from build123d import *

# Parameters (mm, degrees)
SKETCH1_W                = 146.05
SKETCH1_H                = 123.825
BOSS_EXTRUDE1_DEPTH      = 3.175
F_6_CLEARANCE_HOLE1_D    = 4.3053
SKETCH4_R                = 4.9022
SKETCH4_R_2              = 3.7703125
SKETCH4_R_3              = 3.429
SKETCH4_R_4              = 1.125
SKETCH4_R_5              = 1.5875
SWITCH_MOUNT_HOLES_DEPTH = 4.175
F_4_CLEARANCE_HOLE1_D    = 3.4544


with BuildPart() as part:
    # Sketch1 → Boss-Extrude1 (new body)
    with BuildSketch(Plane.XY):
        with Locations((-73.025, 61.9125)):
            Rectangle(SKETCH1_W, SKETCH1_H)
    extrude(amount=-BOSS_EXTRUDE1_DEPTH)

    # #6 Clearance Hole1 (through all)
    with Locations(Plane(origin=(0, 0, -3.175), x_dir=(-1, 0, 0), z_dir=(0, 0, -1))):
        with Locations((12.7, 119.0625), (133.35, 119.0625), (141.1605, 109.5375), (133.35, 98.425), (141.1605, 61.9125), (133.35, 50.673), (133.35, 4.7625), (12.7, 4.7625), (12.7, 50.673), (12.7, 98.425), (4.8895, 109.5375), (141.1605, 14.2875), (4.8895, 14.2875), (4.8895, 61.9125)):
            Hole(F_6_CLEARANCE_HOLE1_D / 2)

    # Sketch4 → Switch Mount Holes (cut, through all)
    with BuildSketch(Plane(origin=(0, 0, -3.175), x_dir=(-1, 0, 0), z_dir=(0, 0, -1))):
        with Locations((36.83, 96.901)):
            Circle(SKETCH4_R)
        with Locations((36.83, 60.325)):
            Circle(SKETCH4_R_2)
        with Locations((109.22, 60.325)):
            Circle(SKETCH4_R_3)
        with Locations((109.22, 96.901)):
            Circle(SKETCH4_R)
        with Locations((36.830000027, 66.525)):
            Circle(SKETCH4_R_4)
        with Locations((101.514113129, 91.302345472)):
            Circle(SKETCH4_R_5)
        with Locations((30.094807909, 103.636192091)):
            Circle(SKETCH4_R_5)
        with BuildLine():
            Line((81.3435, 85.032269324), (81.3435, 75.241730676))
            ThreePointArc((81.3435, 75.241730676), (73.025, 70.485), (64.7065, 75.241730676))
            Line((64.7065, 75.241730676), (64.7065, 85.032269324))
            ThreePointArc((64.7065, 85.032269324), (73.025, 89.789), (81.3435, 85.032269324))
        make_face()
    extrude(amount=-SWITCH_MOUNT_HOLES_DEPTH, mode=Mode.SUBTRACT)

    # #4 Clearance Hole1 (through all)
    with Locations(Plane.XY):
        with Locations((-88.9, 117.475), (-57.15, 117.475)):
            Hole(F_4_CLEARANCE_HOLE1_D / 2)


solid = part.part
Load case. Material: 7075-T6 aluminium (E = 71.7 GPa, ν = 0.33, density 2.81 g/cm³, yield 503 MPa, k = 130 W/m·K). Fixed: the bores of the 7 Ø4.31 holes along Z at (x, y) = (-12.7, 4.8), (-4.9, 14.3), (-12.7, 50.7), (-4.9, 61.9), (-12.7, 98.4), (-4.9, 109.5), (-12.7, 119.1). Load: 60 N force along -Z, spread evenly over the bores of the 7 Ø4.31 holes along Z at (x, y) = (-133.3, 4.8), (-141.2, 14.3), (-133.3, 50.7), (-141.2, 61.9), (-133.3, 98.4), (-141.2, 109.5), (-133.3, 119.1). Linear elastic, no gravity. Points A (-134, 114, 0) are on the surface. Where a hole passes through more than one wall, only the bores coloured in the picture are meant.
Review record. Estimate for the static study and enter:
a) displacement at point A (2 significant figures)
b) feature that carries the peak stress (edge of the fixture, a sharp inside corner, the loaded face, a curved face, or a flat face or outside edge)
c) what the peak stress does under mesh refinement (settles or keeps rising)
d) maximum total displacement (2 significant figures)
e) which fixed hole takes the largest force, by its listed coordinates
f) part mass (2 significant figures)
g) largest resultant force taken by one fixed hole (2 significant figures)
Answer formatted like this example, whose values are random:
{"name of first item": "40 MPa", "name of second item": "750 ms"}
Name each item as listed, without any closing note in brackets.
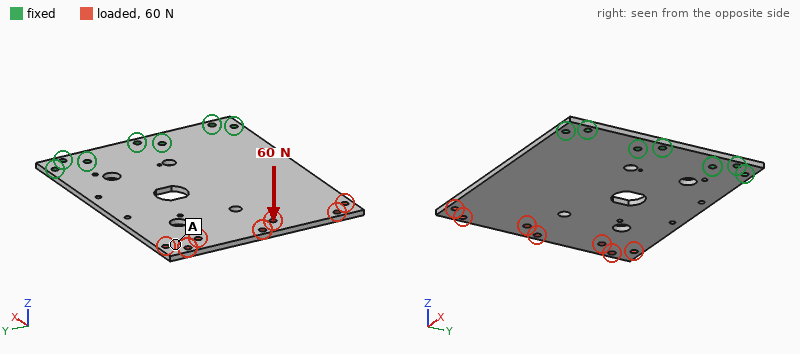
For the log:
{"displacement at point A": "1.7 mm", "feature that carries the peak stress": "edge of the fixture", "what the peak stress does under mesh refinement": "keeps rising", "maximum total displacement": "1.9 mm", "which fixed hole takes the largest force, by its listed coordinates": "(-12.7, 50.7)", "part mass": "150 g", "largest resultant force taken by one fixed hole": "120 N"}
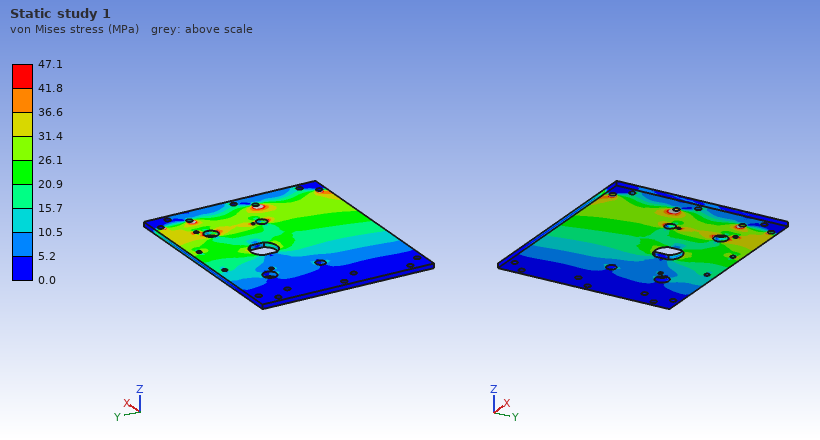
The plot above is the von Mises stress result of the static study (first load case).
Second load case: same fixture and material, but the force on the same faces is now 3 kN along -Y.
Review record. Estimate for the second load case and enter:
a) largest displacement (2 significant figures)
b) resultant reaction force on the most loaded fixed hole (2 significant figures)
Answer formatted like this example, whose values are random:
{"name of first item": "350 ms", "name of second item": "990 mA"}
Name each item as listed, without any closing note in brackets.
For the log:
{"largest displacement": "0.13 mm", "resultant reaction force on the most loaded fixed hole": "2.3 kN"}
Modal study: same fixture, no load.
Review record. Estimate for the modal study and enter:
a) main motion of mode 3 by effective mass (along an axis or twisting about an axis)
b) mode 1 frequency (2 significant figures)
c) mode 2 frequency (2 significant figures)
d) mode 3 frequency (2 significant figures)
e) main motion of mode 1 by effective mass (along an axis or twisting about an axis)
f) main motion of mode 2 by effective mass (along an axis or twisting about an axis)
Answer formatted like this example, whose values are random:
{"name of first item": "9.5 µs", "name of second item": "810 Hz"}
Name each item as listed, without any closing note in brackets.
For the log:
{"main motion of mode 3 by effective mass": "along Z", "mode 1 frequency": "140 Hz", "mode 2 frequency": "380 Hz", "mode 3 frequency": "890 Hz", "main motion of mode 1 by effective mass": "along Z", "main motion of mode 2 by effective mass": "twisting about X"}
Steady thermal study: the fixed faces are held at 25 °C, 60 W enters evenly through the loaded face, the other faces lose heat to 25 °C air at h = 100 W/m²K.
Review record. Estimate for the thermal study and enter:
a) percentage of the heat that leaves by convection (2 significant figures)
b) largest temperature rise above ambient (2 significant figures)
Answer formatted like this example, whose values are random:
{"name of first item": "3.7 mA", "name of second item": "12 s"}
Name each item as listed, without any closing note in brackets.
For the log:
{"percentage of the heat that leaves by convection": "92 %", "largest temperature rise above ambient": "59 K"}
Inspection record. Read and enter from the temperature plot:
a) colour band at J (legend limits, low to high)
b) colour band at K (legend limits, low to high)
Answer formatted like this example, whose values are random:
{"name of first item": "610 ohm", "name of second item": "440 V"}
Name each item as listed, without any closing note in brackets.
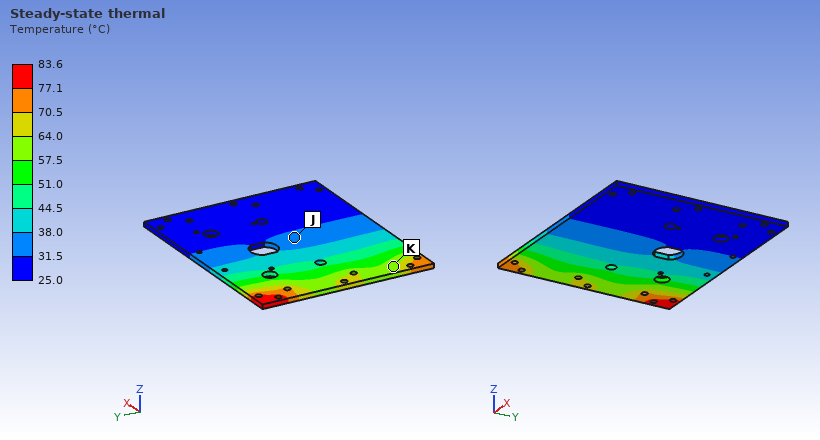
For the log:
{"colour band at J": "31.5 to 38.0 °C", "colour band at K": "57.5 to 64.0 °C"}
